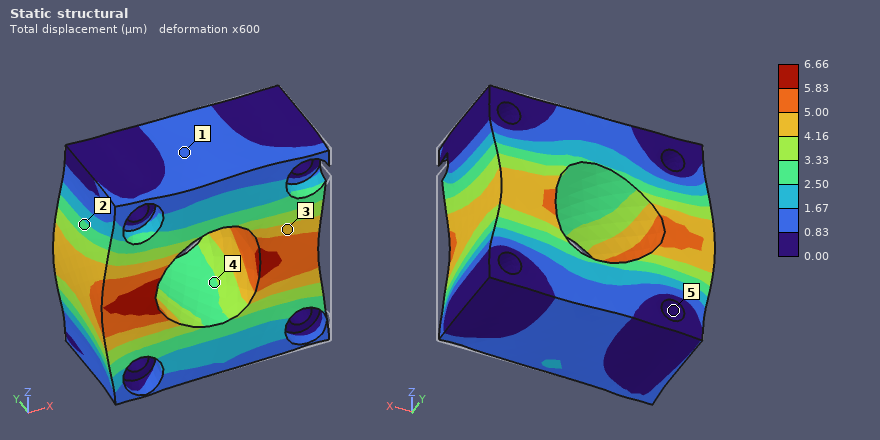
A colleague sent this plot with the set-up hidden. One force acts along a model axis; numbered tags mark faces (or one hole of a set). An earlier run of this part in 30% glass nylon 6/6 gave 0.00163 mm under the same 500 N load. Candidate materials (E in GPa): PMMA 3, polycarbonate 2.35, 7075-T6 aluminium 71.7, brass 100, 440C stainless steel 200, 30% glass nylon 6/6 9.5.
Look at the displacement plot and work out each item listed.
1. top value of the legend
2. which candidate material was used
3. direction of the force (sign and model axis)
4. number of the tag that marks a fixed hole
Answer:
6.66 µm
polycarbonate
-X
5
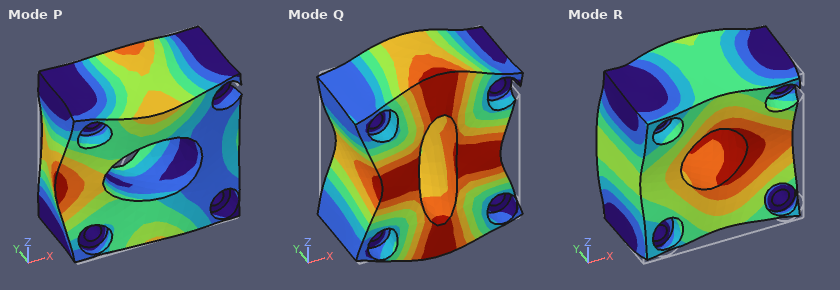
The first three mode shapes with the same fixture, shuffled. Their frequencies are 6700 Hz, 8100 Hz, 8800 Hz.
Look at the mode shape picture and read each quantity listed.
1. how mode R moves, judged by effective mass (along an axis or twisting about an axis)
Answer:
along Y
